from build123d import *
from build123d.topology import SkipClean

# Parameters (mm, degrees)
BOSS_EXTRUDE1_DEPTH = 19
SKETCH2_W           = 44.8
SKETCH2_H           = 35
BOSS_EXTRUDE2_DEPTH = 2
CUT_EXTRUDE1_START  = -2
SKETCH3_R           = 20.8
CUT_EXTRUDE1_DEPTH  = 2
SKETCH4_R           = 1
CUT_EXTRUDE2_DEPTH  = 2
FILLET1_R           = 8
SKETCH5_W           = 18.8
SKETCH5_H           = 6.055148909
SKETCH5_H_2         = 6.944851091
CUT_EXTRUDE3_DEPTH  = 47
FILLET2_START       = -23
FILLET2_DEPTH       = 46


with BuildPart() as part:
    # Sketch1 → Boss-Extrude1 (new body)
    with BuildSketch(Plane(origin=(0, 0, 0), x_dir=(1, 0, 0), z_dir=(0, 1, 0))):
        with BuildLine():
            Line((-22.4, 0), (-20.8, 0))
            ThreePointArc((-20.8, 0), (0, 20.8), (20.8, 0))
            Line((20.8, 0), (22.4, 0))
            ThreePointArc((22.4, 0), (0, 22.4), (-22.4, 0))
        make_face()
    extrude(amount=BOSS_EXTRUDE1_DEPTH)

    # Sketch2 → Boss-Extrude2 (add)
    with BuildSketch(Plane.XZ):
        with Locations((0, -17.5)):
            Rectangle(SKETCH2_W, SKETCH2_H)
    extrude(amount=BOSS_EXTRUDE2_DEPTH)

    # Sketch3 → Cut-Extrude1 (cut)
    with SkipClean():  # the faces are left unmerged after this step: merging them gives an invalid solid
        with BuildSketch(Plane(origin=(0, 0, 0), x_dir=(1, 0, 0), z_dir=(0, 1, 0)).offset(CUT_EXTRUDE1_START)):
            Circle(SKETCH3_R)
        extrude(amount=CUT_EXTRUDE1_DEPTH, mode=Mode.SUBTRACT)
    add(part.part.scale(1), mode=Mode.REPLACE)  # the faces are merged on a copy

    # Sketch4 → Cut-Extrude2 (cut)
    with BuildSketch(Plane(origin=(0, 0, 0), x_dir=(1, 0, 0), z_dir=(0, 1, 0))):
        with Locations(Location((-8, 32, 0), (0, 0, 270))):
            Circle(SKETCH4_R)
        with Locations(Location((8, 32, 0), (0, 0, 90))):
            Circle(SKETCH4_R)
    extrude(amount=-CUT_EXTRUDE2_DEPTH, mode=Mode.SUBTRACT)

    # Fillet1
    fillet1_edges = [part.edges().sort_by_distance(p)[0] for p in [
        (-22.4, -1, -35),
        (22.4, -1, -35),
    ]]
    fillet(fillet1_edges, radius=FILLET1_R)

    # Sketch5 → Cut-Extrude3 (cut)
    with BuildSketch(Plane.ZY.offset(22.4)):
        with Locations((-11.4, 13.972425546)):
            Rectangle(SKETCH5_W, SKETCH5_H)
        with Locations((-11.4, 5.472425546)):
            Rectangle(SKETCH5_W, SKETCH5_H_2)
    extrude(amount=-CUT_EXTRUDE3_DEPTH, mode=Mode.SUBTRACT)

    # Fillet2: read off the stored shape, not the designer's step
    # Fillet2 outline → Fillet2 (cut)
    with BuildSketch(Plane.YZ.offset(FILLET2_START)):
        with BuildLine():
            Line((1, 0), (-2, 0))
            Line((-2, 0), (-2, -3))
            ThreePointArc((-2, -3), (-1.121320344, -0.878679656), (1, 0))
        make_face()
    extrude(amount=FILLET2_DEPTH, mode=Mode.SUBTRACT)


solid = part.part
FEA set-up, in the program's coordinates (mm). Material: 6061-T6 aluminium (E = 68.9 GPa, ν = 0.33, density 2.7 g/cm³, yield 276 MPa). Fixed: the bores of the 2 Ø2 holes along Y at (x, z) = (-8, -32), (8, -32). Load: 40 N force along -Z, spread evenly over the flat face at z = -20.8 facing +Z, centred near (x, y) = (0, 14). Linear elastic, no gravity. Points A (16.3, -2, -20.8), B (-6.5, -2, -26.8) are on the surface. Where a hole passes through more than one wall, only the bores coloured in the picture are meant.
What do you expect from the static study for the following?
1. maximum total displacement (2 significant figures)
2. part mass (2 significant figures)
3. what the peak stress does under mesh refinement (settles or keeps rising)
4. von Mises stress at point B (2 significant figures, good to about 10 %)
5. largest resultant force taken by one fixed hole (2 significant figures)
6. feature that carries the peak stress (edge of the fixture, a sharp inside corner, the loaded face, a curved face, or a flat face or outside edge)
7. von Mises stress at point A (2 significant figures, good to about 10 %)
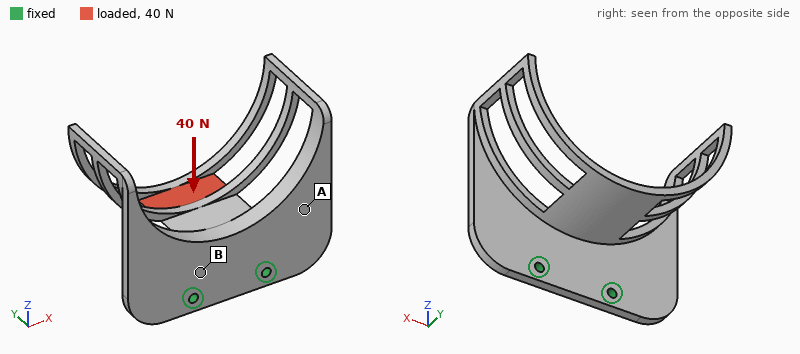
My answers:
0.21 mm
7.2 g
keeps rising
23 MPa
20 N
edge of the fixture
13 MPa
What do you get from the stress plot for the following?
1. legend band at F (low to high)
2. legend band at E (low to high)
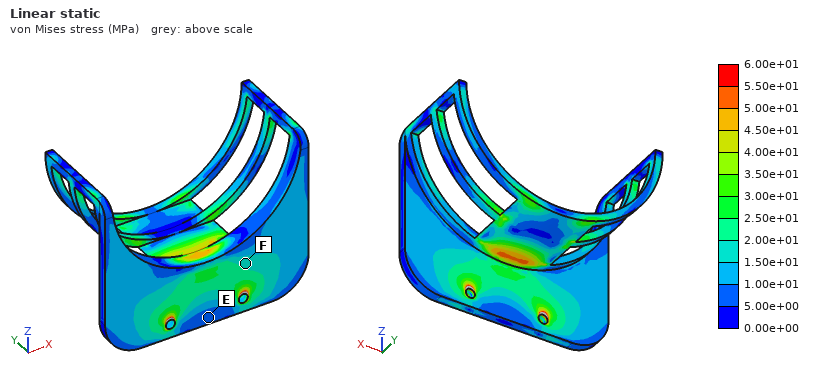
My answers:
1.50e+01 to 2.00e+01 MPa
5.00e+00 to 1.00e+01 MPa
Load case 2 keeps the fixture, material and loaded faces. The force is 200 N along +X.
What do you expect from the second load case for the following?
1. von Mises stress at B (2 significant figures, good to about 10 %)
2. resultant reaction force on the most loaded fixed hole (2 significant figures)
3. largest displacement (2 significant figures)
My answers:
60 MPa
230 N
0.29 mm
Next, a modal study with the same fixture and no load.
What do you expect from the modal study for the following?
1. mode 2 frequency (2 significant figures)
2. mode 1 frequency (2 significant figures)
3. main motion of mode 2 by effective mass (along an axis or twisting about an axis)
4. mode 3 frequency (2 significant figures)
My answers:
1800 Hz
1500 Hz
twisting about Z
2500 Hz
